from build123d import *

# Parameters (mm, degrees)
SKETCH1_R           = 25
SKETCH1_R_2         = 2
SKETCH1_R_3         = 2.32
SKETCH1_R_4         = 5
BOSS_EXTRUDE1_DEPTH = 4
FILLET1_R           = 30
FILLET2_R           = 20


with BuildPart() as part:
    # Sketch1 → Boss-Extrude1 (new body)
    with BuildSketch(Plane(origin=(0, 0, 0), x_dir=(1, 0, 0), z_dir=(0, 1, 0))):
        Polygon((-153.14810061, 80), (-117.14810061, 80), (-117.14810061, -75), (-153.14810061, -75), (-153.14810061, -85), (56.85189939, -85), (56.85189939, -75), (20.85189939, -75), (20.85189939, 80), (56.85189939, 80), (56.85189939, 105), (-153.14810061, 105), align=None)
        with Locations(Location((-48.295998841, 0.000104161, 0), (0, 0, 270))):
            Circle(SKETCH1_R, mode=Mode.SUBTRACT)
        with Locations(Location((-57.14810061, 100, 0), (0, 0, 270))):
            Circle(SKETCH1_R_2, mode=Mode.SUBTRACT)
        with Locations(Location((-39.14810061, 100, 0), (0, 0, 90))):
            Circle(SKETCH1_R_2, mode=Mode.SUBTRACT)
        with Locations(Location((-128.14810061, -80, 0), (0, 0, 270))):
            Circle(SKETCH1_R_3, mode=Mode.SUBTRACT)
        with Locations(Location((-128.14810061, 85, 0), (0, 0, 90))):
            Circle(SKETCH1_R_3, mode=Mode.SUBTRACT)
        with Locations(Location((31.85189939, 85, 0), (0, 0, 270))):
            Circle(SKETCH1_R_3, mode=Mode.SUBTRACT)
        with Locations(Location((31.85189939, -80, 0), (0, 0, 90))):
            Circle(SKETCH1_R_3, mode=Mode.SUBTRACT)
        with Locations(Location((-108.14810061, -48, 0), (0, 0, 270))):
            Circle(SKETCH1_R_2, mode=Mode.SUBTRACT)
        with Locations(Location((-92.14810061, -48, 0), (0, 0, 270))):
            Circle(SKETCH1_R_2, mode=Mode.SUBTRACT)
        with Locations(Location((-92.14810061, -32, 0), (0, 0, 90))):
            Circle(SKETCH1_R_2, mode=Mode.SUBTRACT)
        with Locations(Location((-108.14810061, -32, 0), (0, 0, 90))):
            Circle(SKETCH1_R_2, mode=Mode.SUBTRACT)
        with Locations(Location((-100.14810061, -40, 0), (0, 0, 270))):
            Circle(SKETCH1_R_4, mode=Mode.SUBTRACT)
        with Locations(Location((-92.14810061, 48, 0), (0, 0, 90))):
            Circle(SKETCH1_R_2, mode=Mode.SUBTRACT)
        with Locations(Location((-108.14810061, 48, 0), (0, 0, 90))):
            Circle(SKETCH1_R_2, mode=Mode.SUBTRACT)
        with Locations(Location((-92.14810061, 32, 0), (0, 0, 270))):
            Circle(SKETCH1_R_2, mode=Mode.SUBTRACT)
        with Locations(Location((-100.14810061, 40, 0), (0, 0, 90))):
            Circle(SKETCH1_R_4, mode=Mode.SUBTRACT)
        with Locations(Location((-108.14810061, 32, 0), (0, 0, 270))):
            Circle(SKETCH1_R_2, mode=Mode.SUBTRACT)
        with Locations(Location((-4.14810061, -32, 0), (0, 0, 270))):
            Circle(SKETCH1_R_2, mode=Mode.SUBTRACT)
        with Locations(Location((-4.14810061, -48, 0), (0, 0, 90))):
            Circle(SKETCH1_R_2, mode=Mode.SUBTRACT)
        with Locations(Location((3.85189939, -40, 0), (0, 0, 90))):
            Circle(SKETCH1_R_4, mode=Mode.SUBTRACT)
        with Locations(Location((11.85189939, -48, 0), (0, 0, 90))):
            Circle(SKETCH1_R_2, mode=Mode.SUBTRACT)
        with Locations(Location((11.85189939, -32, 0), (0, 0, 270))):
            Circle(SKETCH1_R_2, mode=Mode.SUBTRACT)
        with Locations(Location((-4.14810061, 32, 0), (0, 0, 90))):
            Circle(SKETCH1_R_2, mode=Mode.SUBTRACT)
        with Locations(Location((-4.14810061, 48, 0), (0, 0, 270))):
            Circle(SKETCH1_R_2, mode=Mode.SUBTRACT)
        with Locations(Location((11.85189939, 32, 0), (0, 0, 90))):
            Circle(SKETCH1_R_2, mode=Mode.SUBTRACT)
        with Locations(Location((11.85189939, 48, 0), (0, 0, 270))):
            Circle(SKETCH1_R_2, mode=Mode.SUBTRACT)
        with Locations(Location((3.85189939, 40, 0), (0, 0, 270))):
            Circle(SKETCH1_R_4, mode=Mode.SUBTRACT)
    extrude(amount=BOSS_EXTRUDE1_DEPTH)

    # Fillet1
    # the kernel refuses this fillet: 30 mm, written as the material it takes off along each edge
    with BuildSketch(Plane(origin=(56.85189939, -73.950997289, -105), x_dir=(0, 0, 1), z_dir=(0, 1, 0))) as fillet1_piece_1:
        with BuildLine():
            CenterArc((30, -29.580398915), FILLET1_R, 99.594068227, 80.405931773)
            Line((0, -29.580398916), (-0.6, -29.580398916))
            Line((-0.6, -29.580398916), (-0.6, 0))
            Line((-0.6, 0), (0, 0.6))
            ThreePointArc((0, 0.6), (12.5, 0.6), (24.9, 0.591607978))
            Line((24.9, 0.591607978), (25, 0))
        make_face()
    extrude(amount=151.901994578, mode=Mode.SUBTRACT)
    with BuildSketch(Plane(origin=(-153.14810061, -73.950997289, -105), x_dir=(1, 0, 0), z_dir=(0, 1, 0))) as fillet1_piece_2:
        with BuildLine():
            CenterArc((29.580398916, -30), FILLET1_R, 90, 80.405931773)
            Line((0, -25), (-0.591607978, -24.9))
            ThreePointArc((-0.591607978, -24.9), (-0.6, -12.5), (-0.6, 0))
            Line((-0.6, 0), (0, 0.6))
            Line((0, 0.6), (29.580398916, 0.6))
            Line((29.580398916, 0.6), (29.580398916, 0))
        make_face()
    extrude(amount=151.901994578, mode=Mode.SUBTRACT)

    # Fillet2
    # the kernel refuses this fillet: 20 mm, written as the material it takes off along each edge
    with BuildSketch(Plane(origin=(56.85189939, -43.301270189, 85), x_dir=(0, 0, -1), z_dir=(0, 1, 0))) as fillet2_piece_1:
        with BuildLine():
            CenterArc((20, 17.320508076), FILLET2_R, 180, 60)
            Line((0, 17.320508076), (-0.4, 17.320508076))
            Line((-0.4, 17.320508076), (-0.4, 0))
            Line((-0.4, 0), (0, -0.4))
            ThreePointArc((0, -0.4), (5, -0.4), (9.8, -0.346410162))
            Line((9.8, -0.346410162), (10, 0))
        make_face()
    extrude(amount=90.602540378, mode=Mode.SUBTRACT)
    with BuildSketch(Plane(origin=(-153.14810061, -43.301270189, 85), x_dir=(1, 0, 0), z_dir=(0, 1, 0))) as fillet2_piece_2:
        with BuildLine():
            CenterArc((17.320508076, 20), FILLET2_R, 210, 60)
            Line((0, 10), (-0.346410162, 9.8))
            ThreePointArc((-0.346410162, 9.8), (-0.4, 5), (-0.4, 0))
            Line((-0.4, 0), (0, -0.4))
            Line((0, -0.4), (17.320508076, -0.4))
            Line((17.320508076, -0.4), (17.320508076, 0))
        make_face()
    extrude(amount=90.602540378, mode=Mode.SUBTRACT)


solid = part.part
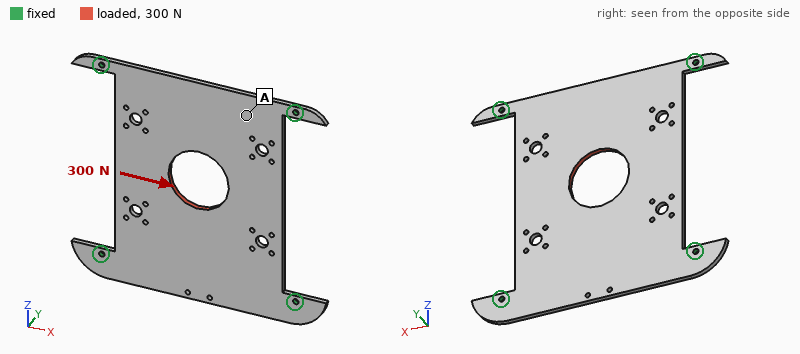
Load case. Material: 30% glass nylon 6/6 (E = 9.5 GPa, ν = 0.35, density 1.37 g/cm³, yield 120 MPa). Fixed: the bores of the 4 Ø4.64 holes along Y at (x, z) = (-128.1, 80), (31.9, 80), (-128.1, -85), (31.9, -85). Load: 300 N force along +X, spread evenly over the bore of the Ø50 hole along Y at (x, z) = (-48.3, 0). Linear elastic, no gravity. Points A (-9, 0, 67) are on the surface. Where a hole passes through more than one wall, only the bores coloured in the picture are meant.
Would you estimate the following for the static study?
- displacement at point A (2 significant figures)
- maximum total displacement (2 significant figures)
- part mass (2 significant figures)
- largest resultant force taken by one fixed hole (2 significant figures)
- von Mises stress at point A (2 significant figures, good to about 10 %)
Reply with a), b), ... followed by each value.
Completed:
a) 6.3 µm
b) 14 µm
c) 140 g
d) 79 N
e) 0.59 MPa
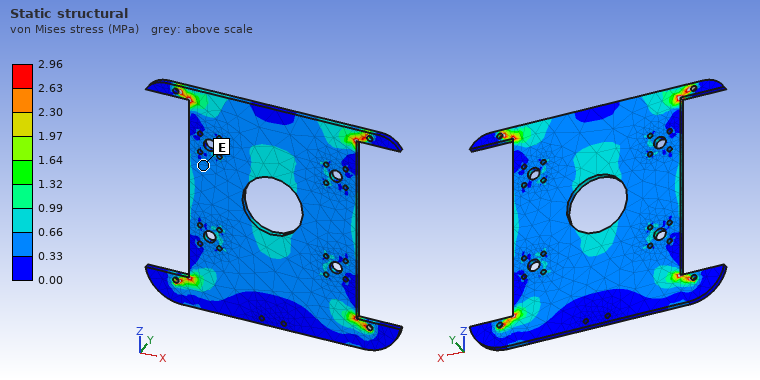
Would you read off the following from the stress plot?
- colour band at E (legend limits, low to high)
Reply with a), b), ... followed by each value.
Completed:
a) 0.33 to 0.66 MPa
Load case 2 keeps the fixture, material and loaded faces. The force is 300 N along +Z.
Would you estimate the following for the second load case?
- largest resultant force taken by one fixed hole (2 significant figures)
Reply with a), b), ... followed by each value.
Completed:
a) 92 N
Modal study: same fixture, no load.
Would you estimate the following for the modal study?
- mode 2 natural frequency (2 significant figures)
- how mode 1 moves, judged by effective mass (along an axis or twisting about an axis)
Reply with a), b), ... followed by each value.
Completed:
a) 390 Hz
b) along Y
